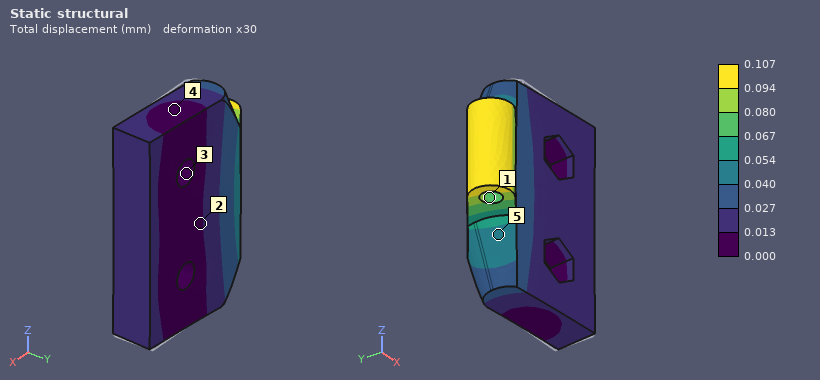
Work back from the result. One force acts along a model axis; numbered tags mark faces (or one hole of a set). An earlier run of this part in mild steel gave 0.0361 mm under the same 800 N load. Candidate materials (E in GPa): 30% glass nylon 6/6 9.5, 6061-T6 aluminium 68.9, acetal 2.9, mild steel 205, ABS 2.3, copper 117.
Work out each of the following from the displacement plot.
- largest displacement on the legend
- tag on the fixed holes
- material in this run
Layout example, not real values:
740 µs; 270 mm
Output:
0.107 mm; 3; 6061-T6 aluminium
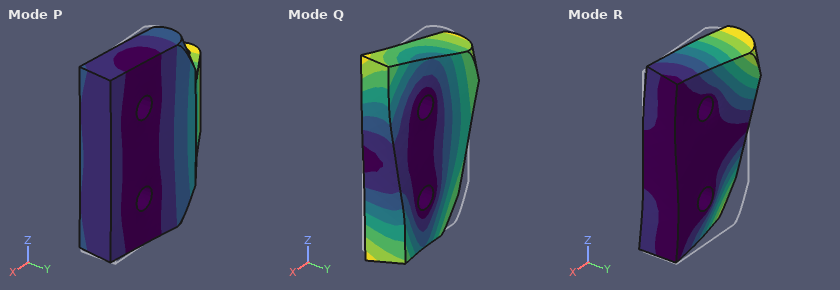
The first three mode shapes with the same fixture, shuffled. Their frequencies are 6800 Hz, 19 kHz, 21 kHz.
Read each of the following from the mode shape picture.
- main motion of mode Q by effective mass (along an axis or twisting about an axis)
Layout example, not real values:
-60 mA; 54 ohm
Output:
along Z
